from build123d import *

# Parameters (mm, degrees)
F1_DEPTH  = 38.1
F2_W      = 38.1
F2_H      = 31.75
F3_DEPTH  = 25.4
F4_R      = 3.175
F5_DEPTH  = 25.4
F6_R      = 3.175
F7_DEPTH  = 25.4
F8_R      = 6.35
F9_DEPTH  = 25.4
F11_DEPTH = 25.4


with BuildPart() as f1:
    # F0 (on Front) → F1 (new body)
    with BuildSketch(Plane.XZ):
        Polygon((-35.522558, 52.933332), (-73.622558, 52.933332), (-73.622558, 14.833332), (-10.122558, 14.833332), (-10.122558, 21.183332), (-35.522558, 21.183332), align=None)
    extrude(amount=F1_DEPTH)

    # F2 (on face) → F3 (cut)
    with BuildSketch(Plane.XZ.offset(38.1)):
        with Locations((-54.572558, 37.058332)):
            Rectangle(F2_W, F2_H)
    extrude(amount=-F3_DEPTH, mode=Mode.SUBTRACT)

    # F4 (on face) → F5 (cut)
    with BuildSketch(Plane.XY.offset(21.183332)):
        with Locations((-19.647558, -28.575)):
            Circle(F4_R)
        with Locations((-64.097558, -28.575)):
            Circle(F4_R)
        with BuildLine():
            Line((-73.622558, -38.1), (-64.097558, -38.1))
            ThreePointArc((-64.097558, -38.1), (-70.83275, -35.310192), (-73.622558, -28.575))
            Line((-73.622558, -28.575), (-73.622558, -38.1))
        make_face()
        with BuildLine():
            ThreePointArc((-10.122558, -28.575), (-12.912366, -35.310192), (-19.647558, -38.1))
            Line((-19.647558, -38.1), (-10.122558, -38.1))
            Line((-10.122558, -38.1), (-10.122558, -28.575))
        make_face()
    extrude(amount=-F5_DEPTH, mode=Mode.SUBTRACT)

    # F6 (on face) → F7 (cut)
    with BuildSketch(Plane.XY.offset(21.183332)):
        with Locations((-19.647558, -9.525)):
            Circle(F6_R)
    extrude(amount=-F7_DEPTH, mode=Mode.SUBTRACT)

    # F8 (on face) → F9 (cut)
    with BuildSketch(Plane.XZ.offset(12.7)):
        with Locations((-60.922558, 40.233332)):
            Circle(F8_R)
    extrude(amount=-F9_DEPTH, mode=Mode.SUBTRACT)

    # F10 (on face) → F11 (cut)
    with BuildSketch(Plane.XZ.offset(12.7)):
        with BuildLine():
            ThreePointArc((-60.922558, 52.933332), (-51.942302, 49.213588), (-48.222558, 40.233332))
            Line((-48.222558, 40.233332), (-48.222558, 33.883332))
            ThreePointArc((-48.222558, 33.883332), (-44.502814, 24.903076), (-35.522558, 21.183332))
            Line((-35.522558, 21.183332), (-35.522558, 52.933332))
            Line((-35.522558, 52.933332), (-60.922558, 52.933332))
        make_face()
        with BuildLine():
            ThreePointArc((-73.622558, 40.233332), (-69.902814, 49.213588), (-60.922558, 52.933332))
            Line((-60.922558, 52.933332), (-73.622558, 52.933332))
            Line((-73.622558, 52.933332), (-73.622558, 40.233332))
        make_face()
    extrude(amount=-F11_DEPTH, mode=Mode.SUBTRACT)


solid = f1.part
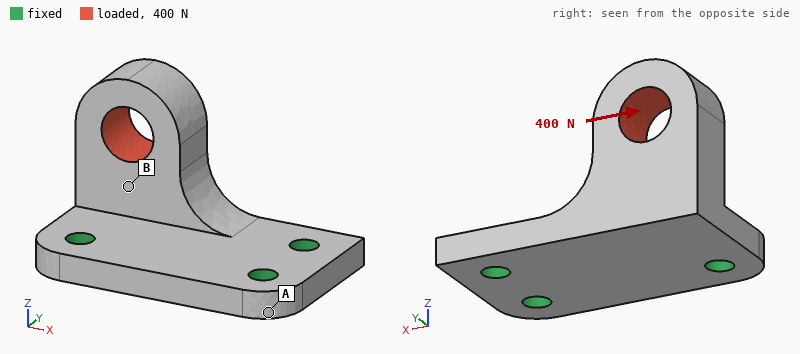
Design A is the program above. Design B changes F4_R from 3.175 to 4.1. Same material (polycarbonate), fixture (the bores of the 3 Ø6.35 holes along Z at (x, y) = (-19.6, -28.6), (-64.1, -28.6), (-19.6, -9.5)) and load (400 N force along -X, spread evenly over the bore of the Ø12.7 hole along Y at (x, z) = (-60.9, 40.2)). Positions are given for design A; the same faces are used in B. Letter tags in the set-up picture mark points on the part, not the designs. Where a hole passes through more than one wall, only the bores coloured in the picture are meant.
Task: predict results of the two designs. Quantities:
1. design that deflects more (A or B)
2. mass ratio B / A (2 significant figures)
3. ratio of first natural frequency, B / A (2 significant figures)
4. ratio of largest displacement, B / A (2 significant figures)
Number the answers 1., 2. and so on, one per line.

1. A
2. 0.99
3. 1.0
4. 0.90
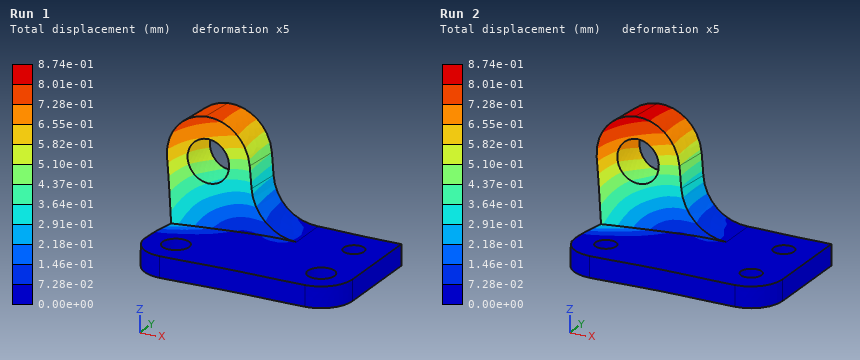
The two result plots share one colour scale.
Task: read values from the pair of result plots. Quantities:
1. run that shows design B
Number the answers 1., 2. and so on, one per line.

1. Run 1
